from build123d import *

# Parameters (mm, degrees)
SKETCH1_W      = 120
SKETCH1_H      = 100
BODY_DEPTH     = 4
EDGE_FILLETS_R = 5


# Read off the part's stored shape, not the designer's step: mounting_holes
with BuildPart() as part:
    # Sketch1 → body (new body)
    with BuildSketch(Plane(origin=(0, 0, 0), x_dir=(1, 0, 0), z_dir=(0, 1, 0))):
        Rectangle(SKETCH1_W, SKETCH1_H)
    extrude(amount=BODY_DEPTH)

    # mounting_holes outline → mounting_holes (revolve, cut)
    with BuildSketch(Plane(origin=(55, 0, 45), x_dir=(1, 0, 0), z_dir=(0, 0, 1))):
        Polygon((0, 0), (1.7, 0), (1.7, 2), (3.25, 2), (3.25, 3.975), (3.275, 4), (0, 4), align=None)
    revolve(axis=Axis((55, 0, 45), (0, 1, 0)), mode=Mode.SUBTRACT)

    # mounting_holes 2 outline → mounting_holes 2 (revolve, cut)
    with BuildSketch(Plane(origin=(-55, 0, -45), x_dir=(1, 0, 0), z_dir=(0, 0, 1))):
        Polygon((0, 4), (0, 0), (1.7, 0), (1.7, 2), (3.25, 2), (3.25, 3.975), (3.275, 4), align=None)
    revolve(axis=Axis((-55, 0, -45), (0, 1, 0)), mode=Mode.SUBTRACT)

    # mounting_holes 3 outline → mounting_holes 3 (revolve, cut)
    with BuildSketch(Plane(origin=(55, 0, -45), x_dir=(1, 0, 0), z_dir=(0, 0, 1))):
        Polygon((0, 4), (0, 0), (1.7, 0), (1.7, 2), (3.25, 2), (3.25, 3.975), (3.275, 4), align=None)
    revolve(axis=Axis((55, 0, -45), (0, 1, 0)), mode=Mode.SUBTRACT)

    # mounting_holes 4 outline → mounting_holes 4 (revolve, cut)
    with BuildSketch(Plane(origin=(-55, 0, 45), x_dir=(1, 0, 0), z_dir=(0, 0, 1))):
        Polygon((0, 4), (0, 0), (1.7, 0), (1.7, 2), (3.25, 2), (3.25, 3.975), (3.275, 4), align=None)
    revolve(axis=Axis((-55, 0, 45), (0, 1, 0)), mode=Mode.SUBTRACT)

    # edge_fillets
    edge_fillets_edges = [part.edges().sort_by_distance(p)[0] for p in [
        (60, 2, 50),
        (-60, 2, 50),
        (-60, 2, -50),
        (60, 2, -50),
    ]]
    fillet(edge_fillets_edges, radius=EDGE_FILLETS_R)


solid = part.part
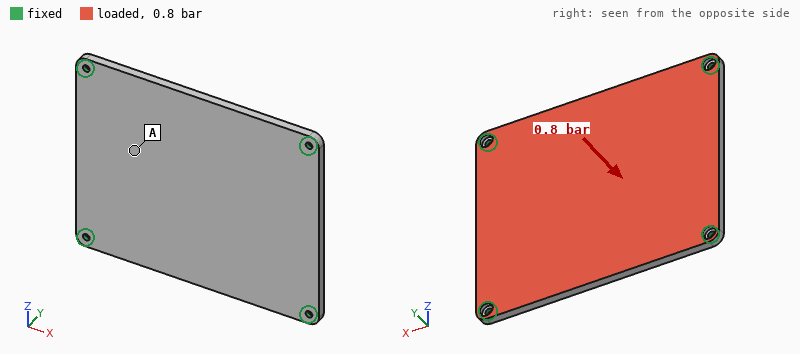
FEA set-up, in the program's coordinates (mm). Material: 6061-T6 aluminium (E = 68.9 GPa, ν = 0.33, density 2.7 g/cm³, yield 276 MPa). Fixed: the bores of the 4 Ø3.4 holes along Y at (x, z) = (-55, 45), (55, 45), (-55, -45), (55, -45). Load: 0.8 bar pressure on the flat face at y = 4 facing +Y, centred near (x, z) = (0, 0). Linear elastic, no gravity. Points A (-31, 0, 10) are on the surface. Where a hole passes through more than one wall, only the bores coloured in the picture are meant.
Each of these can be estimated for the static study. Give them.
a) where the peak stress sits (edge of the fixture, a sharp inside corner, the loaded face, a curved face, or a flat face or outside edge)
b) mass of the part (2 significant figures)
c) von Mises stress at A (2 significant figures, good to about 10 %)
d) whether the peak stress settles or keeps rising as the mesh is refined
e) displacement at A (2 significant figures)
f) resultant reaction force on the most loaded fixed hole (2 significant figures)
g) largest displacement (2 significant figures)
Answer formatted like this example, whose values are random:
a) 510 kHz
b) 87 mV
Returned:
a) edge of the fixture
b) 130 g
c) 15 MPa
d) keeps rising
e) 0.18 mm
f) 550 N
g) 0.24 mm
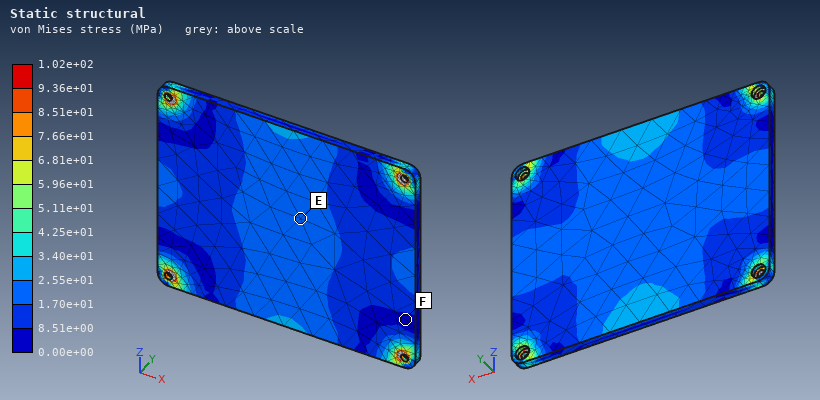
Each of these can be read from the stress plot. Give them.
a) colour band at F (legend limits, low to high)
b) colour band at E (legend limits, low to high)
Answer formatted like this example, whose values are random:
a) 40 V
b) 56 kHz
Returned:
a) 0.00e+00 to 8.51e+00 MPa
b) 1.70e+01 to 2.55e+01 MPa
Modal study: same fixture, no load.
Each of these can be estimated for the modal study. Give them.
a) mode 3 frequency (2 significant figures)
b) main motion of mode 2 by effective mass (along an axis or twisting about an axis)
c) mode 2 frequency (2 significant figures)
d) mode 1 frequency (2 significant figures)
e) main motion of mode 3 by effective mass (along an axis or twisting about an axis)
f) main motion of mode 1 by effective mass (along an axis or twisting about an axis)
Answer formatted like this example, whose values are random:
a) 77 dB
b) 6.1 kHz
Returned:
a) 2200 Hz
b) twisting about X
c) 1800 Hz
d) 1000 Hz
e) twisting about Z
f) along Y
